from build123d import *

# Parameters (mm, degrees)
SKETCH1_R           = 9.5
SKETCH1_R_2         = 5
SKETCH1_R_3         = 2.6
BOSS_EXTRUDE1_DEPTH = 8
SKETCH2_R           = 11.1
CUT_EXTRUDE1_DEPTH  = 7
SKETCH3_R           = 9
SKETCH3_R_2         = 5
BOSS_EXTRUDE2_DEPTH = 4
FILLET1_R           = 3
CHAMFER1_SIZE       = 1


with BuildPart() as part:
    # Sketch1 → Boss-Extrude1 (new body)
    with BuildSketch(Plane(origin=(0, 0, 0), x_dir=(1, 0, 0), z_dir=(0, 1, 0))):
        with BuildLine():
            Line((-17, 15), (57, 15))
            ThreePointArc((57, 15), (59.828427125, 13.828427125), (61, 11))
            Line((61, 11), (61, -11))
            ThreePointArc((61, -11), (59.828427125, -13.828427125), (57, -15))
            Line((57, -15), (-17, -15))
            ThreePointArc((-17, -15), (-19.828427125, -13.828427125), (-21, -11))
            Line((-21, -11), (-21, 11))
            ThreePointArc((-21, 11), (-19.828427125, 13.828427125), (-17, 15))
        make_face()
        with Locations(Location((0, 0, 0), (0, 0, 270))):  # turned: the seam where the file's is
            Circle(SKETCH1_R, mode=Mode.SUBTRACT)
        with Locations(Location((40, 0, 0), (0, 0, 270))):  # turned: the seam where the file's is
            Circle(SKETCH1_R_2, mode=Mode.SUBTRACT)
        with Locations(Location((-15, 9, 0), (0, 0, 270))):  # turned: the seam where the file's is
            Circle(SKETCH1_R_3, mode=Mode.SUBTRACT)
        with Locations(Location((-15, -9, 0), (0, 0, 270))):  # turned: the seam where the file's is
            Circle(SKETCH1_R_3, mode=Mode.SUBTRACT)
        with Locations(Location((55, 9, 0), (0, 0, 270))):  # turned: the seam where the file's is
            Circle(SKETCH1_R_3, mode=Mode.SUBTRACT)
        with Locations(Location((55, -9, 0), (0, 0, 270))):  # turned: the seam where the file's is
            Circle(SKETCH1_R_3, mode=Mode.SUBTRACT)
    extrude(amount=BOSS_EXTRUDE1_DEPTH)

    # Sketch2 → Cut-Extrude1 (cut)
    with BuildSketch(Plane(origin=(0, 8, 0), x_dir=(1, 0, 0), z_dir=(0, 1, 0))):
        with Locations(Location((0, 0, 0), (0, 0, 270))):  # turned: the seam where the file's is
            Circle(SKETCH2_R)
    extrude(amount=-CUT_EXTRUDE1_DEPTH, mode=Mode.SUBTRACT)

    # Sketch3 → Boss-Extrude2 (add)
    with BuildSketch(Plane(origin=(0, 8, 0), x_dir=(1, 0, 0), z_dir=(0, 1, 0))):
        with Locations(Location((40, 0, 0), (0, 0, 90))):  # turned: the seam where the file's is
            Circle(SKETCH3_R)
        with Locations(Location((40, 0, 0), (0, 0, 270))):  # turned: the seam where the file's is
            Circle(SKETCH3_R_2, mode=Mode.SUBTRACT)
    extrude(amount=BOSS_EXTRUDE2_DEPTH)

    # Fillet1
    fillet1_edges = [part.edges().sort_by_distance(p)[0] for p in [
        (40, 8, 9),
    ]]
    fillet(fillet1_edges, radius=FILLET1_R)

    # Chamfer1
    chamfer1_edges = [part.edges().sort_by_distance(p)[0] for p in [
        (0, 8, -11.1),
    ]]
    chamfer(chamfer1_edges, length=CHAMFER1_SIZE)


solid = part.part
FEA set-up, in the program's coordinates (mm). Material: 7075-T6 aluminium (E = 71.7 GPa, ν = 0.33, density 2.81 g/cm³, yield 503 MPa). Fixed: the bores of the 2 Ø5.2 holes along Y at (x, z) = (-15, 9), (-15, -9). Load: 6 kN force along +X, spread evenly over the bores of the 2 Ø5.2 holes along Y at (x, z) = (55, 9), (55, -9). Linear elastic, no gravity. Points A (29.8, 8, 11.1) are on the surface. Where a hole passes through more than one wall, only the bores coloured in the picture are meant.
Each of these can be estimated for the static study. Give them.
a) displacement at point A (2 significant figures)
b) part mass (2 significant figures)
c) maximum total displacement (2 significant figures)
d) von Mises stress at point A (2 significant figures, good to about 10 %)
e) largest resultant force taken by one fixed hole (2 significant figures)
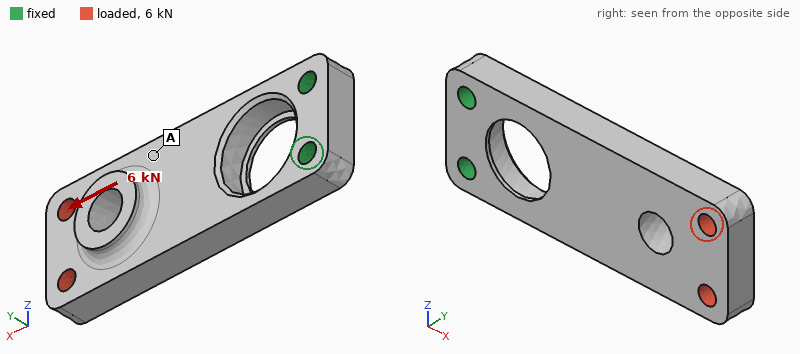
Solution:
55 µm
45 g
76 µm
30 MPa
3.0 kN
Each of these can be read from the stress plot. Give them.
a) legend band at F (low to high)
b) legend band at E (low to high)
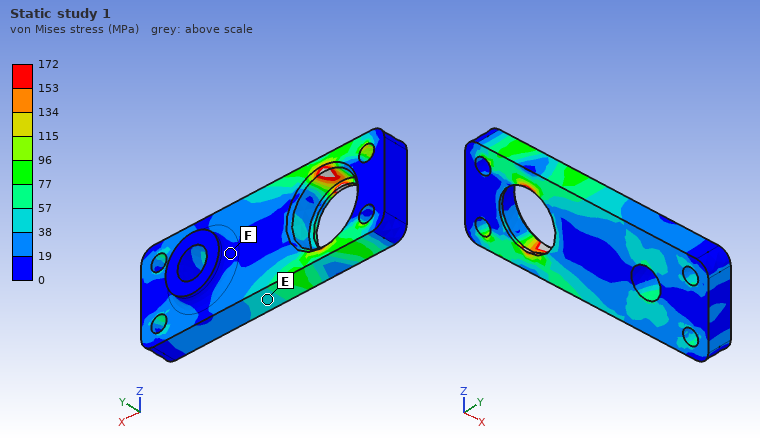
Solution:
0 to 19 MPa
38 to 57 MPa
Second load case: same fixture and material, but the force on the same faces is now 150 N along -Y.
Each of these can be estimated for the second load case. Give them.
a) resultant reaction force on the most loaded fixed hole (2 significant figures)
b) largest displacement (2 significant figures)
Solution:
78 N
0.46 mm
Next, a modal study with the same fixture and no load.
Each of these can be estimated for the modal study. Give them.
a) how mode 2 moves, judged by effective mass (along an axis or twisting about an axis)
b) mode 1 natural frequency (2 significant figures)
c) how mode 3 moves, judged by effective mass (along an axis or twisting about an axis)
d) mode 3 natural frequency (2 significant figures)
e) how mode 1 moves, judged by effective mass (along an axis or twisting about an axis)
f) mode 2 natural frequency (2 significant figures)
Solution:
along Z
770 Hz
twisting about X
4200 Hz
along Y
2600 Hz
